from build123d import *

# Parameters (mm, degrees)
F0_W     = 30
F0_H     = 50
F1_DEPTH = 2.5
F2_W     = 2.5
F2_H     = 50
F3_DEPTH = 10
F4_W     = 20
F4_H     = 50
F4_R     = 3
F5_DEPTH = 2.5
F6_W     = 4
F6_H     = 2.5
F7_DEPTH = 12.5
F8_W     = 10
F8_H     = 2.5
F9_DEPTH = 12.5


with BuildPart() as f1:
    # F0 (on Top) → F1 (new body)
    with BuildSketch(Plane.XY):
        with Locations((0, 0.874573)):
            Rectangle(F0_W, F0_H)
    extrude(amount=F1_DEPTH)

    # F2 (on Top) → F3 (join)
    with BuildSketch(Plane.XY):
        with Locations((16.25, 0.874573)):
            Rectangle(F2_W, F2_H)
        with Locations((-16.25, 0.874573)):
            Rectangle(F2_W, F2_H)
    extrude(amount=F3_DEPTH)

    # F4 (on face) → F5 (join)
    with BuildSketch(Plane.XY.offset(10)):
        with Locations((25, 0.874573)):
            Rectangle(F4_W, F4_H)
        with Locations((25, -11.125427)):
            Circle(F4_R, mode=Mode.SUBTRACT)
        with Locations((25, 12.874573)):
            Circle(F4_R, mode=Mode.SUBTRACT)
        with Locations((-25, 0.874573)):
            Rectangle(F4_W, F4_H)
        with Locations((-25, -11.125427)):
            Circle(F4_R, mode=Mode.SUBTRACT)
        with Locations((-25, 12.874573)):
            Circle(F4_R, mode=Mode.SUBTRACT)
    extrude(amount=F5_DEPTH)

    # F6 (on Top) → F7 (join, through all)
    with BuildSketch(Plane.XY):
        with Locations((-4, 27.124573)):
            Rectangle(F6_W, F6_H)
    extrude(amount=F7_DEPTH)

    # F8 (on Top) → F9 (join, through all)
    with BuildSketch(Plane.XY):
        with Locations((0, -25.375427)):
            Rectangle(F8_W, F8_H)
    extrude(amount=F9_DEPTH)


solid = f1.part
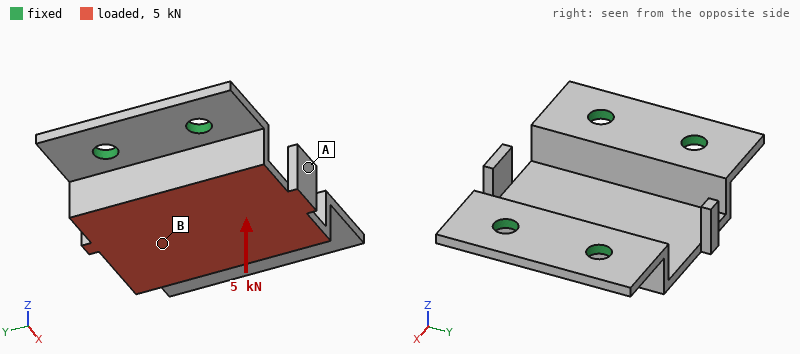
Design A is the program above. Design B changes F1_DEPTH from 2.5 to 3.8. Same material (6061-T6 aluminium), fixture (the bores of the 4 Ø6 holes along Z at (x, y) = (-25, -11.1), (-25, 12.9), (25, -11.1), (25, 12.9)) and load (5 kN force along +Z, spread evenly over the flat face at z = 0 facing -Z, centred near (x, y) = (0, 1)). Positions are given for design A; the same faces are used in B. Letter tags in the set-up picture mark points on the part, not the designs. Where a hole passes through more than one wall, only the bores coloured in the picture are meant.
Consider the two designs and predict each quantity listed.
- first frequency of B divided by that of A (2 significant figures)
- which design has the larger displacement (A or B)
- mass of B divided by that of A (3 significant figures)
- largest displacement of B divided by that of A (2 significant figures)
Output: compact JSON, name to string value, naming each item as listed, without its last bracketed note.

{"first frequency of B divided by that of A": "1.1", "which design has the larger displacement": "A", "mass of B divided by that of A": "1.17", "largest displacement of B divided by that of A": "0.50"}
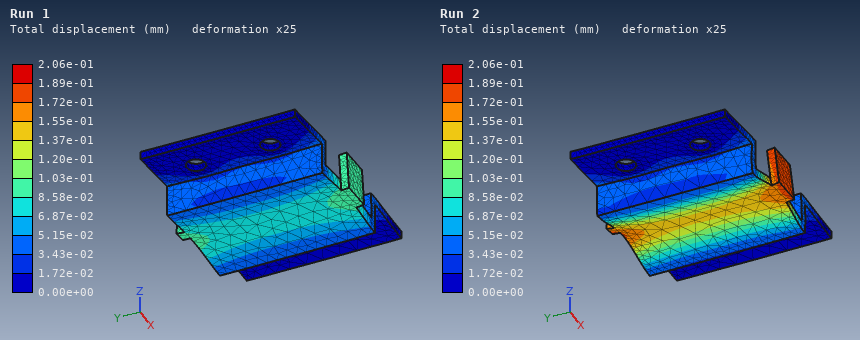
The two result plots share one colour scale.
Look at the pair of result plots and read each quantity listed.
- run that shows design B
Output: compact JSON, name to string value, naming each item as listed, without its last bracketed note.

{"run that shows design B": "Run 1"}
